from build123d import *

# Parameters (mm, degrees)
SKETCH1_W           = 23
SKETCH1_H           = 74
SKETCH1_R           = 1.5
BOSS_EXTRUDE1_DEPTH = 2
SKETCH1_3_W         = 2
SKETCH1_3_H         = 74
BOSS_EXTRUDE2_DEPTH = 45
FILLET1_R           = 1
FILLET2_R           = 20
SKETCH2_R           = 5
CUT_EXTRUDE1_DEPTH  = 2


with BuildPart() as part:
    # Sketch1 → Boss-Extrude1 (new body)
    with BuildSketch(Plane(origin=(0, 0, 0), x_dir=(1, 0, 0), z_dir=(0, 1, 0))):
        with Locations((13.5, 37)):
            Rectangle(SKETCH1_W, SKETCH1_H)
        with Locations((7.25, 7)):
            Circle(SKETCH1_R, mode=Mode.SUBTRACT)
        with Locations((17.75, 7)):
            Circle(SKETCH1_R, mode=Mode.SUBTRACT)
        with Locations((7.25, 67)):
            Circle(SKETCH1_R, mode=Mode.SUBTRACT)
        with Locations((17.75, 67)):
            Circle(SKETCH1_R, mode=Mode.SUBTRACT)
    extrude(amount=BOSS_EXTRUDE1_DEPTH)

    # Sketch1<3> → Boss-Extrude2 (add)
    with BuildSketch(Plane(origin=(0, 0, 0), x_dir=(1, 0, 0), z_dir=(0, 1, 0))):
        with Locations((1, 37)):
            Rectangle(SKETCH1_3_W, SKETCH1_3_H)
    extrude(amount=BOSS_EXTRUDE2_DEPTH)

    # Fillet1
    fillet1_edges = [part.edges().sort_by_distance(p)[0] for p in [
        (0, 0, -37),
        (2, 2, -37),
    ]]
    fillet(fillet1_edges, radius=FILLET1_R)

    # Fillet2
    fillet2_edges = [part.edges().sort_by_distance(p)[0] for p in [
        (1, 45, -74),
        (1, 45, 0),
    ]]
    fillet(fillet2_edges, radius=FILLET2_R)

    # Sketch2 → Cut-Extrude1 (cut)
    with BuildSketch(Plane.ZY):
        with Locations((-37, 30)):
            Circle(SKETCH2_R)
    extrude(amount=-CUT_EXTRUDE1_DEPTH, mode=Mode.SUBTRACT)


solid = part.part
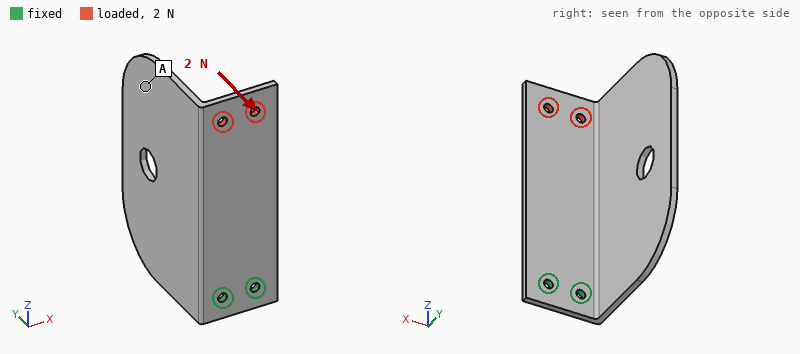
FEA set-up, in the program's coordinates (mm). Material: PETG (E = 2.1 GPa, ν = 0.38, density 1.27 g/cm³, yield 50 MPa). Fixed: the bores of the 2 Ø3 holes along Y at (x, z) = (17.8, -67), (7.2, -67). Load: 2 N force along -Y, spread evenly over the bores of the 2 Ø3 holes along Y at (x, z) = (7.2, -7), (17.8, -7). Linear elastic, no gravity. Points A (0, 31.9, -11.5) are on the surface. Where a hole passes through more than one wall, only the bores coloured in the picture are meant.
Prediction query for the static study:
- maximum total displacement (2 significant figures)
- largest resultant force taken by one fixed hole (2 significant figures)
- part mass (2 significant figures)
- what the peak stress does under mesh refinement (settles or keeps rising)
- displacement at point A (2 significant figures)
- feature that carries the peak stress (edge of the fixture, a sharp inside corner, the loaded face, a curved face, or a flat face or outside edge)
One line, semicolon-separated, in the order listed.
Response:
0.91 mm; 1.1 N; 12 g; keeps rising; 0.71 mm; edge of the fixture
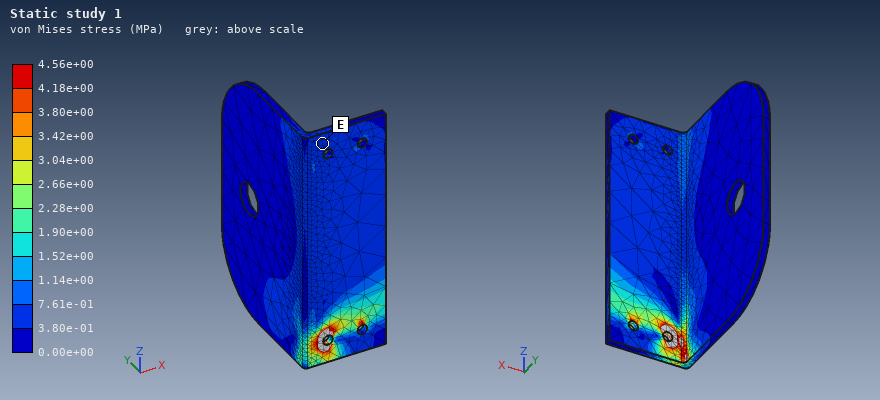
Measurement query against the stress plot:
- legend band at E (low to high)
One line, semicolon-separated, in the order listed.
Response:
3.80e-01 to 7.61e-01 MPa
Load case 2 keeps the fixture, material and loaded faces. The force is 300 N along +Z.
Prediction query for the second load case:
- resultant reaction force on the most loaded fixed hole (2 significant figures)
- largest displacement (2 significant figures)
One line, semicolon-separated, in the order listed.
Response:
150 N; 0.27 mm
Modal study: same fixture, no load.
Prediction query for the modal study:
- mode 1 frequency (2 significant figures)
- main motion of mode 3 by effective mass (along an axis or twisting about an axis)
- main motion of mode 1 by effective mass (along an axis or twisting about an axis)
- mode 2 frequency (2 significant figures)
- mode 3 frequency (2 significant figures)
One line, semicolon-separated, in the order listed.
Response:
110 Hz; twisting about Y; along Y; 140 Hz; 350 Hz
